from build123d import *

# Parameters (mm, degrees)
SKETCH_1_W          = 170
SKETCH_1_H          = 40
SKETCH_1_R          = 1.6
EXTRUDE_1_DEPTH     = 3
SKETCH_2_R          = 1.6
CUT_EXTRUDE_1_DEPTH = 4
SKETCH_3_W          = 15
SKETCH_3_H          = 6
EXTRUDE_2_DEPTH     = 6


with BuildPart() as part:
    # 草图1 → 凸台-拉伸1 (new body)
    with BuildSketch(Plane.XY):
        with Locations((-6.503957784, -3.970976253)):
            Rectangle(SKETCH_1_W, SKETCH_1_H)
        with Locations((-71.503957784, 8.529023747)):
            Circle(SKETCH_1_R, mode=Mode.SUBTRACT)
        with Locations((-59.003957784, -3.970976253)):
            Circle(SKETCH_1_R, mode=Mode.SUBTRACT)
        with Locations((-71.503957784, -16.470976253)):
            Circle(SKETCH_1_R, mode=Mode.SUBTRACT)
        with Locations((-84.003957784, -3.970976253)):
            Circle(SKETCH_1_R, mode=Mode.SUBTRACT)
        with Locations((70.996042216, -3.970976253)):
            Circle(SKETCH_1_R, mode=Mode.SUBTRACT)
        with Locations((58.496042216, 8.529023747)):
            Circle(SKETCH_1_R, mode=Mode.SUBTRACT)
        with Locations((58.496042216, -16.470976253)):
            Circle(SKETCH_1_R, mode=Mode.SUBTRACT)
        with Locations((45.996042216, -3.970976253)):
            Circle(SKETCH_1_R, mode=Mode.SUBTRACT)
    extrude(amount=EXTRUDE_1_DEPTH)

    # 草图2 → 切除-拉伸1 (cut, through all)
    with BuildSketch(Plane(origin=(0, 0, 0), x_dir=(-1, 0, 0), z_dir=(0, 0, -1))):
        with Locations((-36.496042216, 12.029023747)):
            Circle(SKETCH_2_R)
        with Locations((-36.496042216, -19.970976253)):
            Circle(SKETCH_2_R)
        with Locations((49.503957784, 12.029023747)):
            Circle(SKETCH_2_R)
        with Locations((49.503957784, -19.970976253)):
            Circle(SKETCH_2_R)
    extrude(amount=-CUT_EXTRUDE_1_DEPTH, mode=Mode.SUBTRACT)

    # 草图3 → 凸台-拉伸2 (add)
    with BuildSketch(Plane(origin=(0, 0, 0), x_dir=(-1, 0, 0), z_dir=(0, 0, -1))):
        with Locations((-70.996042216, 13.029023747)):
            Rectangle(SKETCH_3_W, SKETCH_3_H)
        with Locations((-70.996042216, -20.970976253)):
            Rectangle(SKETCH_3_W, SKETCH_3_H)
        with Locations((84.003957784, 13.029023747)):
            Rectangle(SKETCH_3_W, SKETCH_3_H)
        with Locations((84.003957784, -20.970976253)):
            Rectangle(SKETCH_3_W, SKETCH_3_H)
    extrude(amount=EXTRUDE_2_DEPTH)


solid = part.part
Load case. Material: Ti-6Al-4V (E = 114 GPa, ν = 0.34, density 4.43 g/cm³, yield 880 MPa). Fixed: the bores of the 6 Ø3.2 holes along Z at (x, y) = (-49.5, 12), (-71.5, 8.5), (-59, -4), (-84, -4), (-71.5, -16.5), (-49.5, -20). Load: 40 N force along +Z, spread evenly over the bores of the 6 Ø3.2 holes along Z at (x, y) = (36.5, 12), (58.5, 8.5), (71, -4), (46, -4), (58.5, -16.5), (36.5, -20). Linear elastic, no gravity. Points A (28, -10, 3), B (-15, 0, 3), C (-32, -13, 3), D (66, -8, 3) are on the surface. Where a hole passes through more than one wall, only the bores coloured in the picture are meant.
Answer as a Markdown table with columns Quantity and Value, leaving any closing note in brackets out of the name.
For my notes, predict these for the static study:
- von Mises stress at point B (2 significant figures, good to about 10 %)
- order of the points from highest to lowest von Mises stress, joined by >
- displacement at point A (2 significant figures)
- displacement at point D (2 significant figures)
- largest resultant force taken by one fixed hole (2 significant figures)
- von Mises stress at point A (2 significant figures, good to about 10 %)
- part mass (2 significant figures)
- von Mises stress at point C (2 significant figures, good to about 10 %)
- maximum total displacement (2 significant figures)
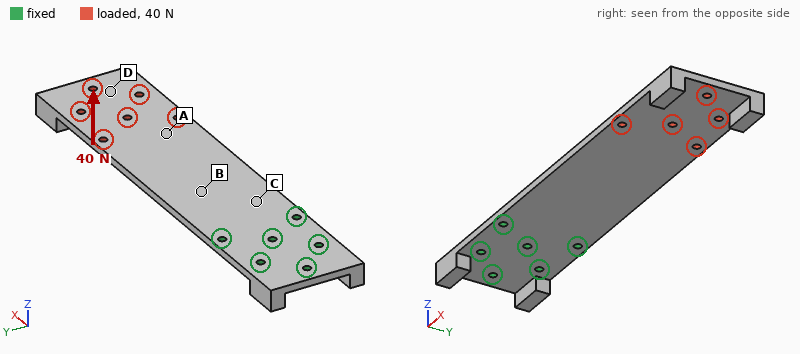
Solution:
| Quantity | Value |
|---|---|
| von Mises stress at point B | 43 MPa |
| order of the points from highest to lowest von Mises stress, joined by > | C > B > A > D |
| displacement at point A | 0.90 mm |
| displacement at point D | 1.6 mm |
| largest resultant force taken by one fixed hole | 78 N |
| von Mises stress at point A | 16 MPa |
| part mass | 99 g |
| von Mises stress at point C | 53 MPa |
| maximum total displacement | 1.9 mm |
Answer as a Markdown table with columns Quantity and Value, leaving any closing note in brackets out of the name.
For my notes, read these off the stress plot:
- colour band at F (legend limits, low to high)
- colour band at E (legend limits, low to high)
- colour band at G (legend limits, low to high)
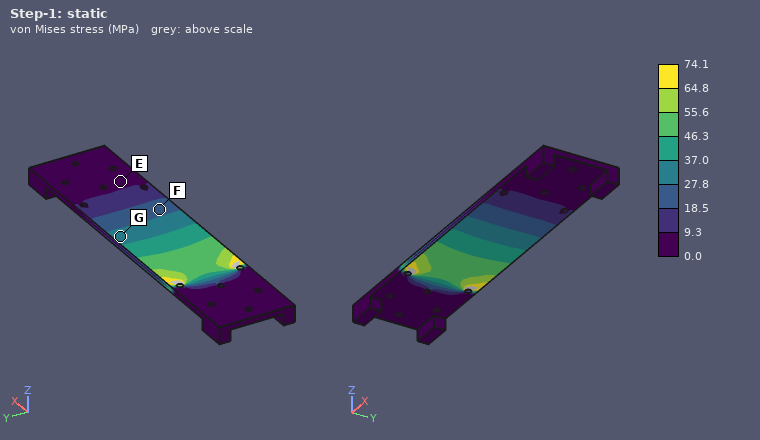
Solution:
| Quantity | Value |
|---|---|
| colour band at F | 18.5 to 27.8 MPa |
| colour band at E | 0.0 to 9.3 MPa |
| colour band at G | 27.8 to 37.0 MPa |
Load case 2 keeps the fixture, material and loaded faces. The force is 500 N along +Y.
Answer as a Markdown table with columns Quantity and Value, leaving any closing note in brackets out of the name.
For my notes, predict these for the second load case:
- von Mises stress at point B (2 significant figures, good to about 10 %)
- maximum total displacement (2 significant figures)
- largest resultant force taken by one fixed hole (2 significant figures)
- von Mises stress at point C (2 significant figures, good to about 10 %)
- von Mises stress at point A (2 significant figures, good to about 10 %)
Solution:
| Quantity | Value |
|---|---|
| von Mises stress at point B | 14 MPa |
| maximum total displacement | 0.15 mm |
| largest resultant force taken by one fixed hole | 1.4 kN |
| von Mises stress at point C | 25 MPa |
| von Mises stress at point A | 11 MPa |
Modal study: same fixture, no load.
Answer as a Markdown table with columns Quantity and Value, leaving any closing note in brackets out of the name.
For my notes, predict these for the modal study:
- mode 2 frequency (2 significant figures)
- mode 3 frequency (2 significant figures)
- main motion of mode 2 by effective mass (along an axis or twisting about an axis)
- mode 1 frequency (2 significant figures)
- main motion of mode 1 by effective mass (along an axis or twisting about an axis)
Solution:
| Quantity | Value |
|---|---|
| mode 2 frequency | 830 Hz |
| mode 3 frequency | 870 Hz |
| main motion of mode 2 by effective mass | twisting about X |
| mode 1 frequency | 130 Hz |
| main motion of mode 1 by effective mass | along Z |
